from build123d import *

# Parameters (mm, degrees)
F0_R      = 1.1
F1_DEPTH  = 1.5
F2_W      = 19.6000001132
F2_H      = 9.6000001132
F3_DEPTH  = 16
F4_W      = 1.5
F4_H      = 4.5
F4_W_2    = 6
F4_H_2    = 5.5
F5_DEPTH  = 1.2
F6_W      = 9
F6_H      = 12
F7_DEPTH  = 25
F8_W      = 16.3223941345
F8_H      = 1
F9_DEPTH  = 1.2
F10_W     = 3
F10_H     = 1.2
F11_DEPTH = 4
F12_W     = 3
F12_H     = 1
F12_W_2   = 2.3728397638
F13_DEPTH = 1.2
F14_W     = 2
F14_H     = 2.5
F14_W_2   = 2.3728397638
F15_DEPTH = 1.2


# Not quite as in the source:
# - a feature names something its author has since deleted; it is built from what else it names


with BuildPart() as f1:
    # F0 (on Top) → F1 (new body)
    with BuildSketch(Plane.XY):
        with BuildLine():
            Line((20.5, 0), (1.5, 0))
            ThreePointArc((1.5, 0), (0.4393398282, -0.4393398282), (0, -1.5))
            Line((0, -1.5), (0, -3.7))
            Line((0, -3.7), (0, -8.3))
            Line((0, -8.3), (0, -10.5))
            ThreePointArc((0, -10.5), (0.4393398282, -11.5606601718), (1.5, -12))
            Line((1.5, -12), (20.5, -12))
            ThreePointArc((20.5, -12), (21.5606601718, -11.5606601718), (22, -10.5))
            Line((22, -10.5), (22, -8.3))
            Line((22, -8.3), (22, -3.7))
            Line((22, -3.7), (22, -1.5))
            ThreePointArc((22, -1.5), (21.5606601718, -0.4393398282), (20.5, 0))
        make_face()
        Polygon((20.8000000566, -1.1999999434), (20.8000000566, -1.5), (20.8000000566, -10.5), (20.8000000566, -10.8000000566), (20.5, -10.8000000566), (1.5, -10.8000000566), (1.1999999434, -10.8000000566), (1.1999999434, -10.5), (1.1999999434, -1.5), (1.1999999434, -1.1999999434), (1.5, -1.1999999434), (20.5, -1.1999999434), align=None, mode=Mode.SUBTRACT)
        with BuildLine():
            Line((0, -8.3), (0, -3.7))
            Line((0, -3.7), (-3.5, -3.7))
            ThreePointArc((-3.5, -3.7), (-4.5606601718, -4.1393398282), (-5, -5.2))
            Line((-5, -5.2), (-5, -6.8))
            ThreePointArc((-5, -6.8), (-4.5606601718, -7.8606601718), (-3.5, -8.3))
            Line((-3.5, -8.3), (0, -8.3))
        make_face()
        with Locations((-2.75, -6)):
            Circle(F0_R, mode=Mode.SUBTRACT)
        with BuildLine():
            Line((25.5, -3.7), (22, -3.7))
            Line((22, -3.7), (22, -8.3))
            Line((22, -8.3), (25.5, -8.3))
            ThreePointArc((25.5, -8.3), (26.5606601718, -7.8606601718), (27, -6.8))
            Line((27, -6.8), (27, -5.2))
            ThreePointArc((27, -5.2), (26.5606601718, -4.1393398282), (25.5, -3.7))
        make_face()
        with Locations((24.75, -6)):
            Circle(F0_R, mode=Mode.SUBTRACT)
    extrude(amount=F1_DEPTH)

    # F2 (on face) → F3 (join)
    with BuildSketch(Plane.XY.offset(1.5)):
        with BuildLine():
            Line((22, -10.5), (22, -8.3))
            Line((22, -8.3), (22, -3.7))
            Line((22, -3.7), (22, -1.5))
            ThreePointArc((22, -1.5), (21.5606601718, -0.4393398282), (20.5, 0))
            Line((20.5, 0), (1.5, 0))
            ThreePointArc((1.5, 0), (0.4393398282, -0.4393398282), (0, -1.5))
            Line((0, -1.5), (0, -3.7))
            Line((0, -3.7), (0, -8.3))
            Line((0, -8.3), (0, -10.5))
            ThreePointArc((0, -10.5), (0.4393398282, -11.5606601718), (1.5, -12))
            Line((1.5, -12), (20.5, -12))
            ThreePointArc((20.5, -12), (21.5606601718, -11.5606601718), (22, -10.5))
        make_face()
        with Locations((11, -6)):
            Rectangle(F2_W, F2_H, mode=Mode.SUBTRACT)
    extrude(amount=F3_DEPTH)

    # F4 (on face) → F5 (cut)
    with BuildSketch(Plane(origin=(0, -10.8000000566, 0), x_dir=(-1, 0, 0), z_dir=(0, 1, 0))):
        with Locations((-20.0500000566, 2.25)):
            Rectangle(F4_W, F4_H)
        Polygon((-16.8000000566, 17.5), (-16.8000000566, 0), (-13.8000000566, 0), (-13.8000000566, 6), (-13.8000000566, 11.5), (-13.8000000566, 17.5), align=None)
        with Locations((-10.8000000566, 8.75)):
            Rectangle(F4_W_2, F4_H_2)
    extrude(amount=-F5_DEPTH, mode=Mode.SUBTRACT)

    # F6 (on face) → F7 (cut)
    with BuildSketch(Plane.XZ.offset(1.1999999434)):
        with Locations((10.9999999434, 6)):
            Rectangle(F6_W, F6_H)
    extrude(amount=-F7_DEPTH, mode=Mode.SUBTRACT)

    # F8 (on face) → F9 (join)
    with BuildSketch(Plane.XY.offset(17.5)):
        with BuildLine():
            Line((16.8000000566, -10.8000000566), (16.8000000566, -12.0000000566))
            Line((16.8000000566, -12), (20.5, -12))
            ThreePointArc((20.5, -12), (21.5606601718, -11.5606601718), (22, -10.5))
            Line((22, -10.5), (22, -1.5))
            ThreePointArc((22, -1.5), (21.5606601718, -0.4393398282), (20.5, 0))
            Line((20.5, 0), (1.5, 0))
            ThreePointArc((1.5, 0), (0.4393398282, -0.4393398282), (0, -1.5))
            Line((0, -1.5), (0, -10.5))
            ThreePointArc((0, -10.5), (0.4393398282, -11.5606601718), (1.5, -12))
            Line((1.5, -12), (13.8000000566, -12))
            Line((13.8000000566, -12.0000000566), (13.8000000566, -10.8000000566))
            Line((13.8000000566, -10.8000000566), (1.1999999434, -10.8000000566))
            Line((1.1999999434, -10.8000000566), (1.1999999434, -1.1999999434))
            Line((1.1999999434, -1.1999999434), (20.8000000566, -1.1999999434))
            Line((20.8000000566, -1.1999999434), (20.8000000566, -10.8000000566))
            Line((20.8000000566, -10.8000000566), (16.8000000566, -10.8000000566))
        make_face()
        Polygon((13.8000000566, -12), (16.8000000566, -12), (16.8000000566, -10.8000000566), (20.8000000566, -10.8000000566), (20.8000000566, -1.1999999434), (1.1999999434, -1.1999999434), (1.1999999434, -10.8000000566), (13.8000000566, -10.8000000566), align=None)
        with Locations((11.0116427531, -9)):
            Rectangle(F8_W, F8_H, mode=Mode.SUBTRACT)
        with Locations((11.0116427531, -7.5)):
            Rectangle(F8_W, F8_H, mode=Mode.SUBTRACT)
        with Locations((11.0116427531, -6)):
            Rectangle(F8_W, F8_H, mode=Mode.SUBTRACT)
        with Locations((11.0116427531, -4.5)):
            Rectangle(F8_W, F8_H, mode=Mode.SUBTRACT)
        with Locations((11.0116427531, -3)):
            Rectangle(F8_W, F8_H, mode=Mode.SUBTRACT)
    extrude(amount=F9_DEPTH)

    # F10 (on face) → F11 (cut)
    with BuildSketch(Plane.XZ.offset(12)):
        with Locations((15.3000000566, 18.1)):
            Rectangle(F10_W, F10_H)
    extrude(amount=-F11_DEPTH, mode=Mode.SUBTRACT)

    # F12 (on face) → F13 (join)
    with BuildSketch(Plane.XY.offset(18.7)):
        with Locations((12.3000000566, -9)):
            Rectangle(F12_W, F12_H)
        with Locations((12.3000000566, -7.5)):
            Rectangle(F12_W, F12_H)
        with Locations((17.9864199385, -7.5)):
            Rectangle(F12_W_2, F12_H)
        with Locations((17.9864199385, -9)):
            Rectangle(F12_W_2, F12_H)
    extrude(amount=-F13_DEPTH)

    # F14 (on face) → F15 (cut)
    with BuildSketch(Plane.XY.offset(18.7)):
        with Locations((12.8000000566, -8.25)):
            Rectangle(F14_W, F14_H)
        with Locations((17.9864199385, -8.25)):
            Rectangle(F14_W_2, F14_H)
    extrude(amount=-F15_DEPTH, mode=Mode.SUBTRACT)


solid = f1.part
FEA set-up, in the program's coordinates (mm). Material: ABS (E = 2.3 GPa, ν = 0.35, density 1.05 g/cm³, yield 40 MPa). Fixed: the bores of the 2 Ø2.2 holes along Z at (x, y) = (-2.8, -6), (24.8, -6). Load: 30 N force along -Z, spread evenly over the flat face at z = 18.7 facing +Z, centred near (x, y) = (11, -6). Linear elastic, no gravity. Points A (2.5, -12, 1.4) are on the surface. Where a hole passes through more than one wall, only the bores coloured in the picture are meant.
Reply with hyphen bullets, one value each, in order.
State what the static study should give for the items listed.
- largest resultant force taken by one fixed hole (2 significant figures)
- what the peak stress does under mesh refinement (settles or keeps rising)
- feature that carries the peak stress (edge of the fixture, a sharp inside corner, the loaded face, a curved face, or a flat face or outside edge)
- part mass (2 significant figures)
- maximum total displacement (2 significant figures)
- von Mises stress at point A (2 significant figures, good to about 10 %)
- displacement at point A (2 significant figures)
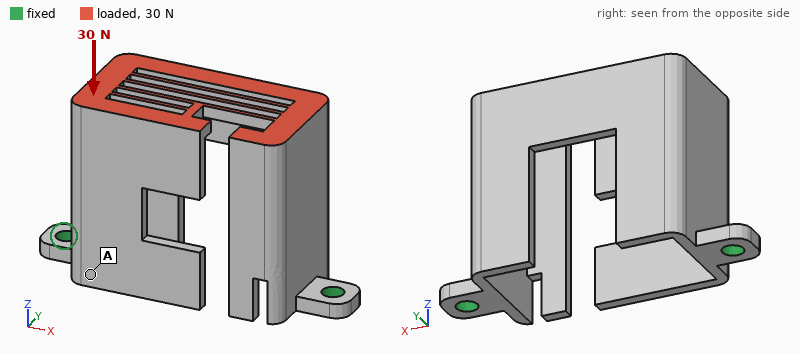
- 16 N
- keeps rising
- edge of the fixture
- 1.4 g
- 0.40 mm
- 1.7 MPa
- 0.10 mm
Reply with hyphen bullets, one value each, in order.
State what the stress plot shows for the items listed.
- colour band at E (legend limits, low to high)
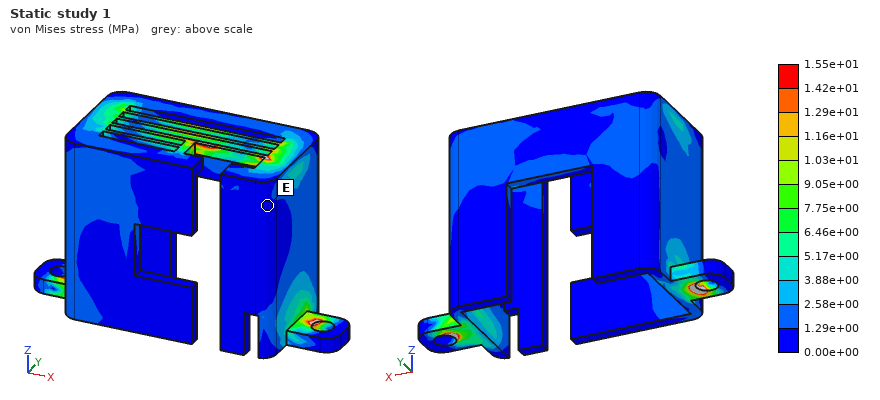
- 0.00e+00 to 1.29e+00 MPa
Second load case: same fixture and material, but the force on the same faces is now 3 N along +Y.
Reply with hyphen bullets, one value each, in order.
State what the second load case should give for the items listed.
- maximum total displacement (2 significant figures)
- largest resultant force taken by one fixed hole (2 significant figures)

- 0.32 mm
- 1.6 N
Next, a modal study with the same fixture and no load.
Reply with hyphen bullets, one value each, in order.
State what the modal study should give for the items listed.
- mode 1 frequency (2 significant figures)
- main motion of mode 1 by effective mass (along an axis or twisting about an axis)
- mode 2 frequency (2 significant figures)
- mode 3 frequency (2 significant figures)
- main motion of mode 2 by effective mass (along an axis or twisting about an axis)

- 690 Hz
- along Y
- 830 Hz
- 1400 Hz
- along X
